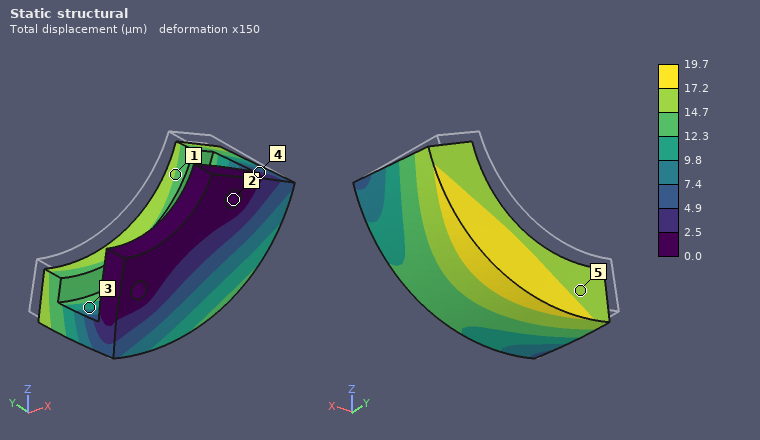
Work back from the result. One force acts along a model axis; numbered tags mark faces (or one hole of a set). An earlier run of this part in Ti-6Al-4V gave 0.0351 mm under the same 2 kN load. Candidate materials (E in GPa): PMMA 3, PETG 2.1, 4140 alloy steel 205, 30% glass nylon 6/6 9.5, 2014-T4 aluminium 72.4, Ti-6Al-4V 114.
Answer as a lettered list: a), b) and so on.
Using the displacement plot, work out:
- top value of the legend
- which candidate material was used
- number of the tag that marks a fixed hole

a) 19.7 µm
b) 4140 alloy steel
c) 2
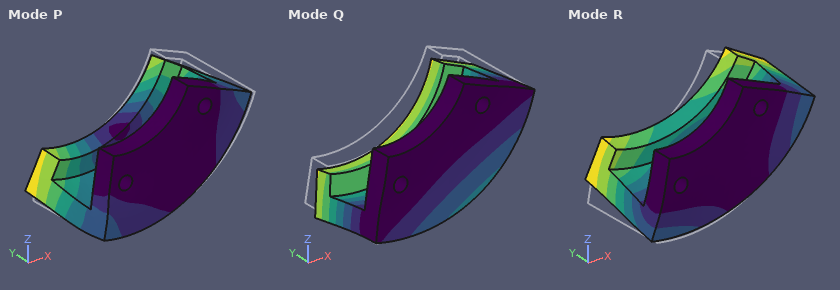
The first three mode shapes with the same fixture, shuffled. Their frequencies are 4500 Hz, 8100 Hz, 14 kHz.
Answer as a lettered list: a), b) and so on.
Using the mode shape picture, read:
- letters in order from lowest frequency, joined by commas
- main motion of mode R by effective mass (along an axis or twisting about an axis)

a) Q, R, P
b) along X
